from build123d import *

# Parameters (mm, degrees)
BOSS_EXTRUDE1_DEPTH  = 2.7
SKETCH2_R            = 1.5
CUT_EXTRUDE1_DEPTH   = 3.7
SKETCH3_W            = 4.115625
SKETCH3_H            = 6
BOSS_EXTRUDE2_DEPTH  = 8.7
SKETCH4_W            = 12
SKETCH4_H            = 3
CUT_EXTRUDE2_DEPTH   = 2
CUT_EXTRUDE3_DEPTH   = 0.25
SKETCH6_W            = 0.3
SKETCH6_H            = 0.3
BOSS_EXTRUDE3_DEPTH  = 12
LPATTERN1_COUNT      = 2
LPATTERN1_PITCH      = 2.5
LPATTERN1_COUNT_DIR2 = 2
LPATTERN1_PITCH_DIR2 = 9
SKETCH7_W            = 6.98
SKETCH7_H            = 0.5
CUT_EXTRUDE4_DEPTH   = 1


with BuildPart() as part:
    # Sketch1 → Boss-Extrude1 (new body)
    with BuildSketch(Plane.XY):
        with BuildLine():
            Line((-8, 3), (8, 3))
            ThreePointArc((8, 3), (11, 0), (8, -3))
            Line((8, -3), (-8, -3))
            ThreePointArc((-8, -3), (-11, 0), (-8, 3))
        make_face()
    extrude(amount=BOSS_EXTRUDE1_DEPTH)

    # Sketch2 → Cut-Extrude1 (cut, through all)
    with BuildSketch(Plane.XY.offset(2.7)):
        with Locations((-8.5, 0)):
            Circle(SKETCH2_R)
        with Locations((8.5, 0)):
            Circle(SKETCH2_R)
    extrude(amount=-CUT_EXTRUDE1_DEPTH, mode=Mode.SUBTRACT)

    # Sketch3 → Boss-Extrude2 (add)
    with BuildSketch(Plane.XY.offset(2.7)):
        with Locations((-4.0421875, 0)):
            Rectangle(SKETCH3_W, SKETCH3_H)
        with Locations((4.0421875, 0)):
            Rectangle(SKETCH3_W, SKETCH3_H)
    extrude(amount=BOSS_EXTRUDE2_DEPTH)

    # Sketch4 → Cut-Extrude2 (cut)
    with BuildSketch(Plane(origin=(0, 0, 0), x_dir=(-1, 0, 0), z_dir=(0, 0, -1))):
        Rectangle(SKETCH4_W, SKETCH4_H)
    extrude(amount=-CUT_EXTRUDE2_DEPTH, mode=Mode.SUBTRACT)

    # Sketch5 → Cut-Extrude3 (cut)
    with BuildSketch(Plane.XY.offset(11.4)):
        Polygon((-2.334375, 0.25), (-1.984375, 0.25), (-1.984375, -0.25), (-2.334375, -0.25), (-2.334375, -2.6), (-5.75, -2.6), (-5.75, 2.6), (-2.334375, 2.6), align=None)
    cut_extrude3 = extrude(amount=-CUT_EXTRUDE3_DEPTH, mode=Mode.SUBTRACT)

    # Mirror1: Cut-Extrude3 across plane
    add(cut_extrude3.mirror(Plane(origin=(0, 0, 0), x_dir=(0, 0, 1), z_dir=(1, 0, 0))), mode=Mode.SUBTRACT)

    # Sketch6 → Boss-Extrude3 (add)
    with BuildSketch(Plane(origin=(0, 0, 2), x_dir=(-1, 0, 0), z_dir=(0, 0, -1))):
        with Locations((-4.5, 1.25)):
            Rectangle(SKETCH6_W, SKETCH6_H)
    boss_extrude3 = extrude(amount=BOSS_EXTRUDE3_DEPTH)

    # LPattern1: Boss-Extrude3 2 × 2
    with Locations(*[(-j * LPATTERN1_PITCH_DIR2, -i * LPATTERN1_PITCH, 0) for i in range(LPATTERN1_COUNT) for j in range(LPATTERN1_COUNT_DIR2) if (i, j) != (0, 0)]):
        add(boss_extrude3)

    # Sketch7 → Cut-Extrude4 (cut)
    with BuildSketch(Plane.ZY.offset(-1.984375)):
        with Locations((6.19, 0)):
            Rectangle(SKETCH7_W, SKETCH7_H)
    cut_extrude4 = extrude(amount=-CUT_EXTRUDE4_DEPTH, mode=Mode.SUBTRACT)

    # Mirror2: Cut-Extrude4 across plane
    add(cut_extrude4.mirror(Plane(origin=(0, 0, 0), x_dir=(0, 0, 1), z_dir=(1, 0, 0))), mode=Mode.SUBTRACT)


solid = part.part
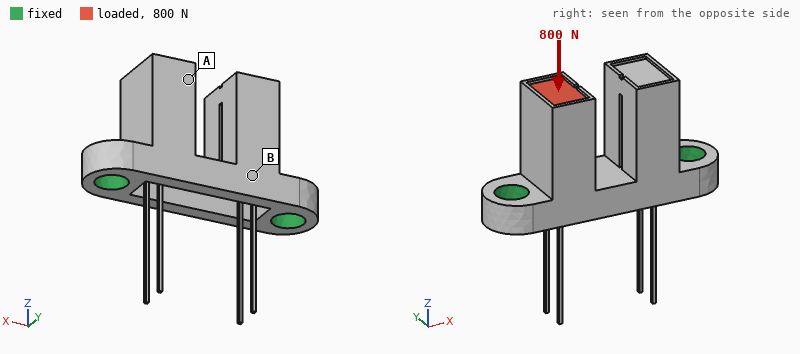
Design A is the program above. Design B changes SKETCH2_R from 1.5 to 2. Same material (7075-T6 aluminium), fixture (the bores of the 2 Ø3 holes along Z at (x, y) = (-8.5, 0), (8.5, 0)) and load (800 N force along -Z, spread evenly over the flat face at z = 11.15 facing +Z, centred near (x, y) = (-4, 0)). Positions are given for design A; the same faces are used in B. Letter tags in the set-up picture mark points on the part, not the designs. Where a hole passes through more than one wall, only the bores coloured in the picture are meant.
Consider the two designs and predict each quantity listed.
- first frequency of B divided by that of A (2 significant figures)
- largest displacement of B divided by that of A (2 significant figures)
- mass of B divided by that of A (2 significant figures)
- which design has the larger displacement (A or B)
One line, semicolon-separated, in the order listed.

1.00; 0.92; 0.95; A
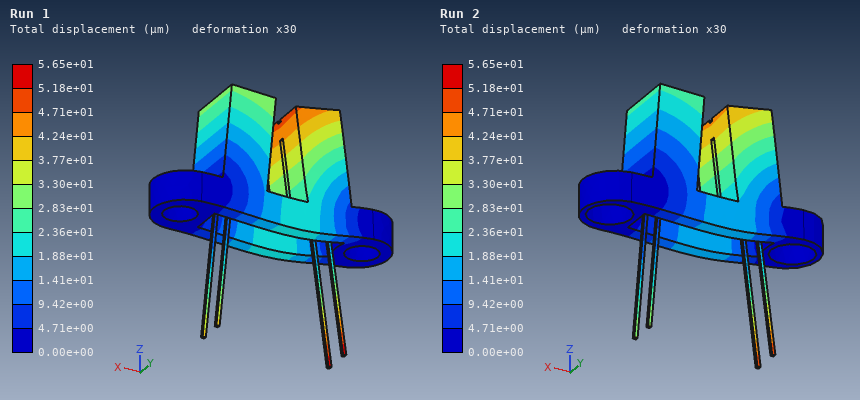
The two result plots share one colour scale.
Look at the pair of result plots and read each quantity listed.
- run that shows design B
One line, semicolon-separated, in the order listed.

Run 2
